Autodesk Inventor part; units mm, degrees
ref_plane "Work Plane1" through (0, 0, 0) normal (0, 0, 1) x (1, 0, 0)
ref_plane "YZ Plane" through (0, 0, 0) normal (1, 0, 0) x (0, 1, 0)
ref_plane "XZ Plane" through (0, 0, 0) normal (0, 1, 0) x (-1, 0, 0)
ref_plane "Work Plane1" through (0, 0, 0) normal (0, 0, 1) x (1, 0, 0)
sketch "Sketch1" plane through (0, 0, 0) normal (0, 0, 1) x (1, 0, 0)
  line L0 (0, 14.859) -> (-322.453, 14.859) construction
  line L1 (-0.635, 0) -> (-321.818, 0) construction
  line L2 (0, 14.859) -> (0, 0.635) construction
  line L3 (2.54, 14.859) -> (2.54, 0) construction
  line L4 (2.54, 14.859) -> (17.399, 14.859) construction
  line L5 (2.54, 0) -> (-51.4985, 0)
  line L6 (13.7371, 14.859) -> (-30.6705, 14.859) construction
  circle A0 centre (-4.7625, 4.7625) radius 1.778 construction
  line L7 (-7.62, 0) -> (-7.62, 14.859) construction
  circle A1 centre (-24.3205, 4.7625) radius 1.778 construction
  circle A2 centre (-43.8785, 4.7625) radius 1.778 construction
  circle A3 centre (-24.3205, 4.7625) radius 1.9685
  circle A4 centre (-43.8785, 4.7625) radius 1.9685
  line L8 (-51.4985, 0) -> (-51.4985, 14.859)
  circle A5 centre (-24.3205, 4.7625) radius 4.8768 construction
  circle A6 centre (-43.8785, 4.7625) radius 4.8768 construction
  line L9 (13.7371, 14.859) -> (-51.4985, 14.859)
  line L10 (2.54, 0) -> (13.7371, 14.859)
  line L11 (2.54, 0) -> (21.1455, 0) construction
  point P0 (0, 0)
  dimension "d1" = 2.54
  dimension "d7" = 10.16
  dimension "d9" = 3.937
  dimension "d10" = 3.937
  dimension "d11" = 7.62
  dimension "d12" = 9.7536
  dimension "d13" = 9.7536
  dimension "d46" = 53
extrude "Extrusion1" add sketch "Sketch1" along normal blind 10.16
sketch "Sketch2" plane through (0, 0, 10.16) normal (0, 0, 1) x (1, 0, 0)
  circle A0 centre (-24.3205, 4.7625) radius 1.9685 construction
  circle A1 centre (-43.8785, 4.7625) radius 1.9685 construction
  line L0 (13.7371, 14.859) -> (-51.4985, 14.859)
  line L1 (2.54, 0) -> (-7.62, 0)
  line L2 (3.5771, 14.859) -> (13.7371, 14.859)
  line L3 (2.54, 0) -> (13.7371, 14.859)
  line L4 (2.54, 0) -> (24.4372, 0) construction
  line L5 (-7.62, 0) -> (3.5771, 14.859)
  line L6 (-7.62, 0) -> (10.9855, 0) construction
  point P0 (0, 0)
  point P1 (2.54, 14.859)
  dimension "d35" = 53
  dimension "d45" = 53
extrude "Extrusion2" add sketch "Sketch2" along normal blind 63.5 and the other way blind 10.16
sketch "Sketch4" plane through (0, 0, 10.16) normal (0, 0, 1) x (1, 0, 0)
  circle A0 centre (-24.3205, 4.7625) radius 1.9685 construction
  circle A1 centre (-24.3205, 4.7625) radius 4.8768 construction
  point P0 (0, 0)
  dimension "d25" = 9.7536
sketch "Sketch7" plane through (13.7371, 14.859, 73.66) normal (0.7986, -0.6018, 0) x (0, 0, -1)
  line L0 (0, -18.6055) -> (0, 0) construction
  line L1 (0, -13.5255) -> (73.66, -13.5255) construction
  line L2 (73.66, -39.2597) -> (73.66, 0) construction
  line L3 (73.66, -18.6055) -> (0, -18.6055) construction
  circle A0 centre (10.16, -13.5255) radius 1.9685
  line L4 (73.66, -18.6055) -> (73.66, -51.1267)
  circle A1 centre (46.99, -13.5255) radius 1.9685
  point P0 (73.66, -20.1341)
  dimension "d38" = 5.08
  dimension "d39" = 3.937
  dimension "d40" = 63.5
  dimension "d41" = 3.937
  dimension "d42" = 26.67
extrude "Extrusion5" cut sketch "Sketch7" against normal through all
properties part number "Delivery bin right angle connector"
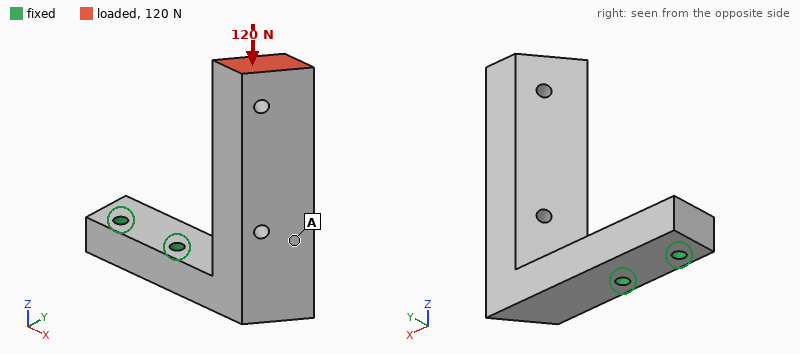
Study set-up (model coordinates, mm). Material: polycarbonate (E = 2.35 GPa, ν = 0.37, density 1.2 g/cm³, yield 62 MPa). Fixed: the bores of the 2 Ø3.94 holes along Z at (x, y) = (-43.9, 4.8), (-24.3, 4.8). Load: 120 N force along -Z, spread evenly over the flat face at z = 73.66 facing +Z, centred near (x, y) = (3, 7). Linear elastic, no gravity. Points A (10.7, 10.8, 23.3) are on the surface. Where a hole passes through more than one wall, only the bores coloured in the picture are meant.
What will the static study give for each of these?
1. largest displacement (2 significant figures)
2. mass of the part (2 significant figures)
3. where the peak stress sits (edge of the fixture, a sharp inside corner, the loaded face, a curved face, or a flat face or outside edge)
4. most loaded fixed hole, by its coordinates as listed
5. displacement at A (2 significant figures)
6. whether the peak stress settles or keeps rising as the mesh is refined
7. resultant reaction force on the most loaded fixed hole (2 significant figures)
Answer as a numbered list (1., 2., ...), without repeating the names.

1. 1.2 mm
2. 22 g
3. edge of the fixture
4. (-24.3, 4.8)
5. 0.52 mm
6. keeps rising
7. 160 N
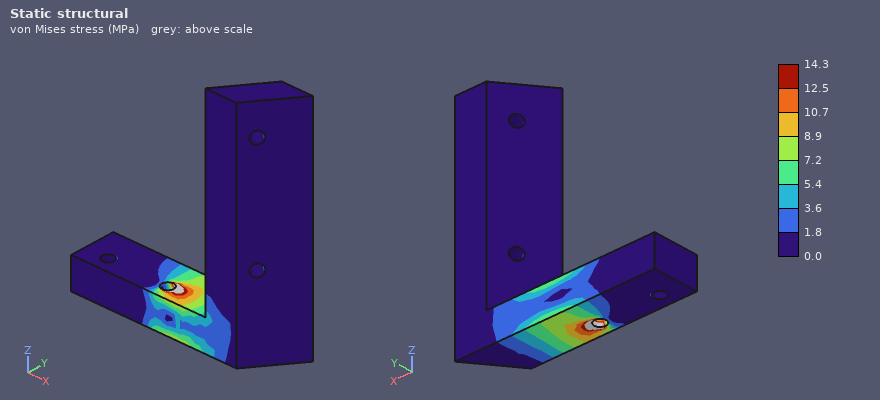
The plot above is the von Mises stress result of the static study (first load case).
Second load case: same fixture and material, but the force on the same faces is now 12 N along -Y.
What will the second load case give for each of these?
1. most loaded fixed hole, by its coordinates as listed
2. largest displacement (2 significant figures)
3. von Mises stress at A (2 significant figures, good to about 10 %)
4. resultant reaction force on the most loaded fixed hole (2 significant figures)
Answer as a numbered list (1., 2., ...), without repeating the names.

1. (-24.3, 4.8)
2. 1.0 mm
3. 1.3 MPa
4. 25 N
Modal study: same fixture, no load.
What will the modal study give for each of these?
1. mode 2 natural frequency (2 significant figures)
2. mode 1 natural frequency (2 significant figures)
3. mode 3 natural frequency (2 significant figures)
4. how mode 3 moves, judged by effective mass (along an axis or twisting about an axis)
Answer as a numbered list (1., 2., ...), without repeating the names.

1. 350 Hz
2. 270 Hz
3. 1200 Hz
4. along Z
